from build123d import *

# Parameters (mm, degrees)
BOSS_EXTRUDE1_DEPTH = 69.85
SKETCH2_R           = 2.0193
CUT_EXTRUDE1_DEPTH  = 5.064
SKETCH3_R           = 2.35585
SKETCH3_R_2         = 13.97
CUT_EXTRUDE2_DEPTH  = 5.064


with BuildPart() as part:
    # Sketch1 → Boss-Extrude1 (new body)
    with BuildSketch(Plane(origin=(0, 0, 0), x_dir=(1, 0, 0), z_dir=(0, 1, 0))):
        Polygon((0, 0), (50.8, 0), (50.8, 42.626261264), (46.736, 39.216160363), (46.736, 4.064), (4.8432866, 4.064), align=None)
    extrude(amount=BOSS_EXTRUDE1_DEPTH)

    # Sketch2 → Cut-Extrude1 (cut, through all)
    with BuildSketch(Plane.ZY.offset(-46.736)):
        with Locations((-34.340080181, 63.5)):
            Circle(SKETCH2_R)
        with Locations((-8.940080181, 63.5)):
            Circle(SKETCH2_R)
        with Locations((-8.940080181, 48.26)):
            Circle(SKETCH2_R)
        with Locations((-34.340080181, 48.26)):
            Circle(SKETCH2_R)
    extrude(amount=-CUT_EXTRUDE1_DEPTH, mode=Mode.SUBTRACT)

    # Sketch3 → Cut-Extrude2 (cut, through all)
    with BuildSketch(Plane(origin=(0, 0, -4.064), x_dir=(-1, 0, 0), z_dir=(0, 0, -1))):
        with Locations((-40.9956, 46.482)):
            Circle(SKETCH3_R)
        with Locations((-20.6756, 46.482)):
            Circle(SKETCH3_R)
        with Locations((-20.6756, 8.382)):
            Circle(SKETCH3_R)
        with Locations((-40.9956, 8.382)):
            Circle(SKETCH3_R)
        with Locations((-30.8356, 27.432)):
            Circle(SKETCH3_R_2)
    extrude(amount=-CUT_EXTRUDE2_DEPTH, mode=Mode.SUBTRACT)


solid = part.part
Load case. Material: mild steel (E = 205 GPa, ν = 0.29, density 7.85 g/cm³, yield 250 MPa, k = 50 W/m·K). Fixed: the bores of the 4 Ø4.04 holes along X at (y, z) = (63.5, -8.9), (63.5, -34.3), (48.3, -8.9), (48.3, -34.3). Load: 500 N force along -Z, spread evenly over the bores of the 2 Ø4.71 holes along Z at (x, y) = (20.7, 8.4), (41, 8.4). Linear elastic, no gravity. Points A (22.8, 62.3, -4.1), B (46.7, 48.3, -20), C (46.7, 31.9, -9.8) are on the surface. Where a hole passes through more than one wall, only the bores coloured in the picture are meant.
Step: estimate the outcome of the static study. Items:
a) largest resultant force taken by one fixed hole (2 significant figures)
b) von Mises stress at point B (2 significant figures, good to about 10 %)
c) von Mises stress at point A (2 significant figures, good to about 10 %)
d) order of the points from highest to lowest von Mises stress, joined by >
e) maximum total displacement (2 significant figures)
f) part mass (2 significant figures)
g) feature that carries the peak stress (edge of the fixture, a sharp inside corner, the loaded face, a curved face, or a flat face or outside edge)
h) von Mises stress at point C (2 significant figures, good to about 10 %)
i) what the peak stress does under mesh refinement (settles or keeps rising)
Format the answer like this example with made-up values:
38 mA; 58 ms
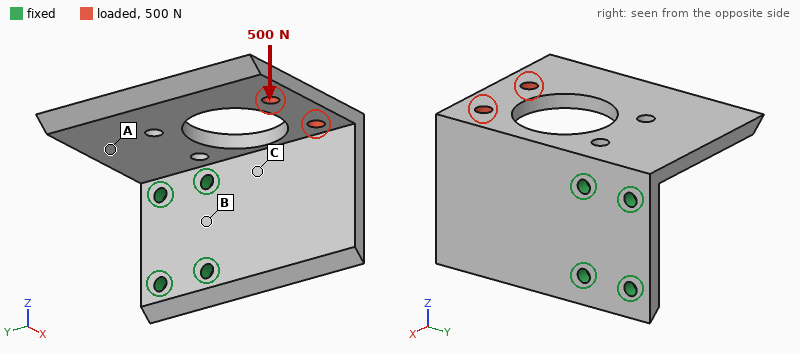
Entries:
720 N; 13 MPa; 29 MPa; C > A > B; 0.26 mm; 170 g; edge of the fixture; 44 MPa; keeps rising
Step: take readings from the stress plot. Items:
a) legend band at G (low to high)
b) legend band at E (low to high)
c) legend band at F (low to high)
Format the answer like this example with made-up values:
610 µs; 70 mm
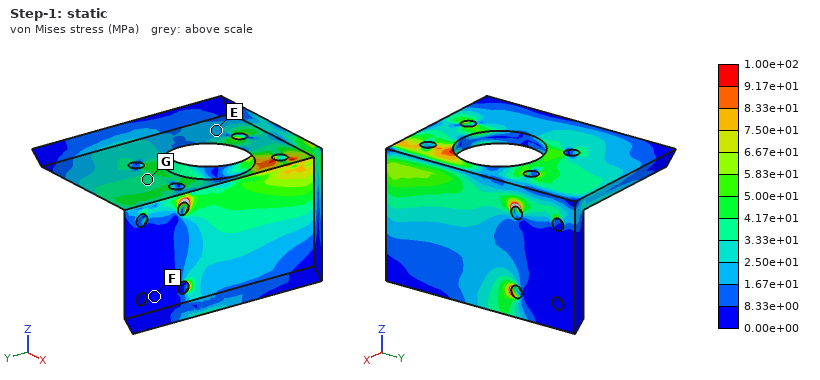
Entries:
3.33e+01 to 4.17e+01 MPa; 1.67e+01 to 2.50e+01 MPa; 0.00e+00 to 8.33e+00 MPa
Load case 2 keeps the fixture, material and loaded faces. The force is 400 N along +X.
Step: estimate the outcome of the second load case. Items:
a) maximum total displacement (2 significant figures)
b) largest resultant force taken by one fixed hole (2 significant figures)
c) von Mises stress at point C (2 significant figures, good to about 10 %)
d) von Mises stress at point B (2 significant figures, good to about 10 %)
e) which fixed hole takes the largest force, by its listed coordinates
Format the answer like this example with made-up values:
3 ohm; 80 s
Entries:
60 µm; 1.2 kN; 12 MPa; 12 MPa; (48.3, -8.9)
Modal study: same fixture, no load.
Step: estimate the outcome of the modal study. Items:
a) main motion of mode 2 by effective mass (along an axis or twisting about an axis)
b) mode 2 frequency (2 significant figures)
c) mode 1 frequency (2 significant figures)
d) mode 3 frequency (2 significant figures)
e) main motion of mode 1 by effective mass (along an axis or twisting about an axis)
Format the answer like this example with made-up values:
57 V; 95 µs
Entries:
along X; 2000 Hz; 1000 Hz; 2100 Hz; along Z
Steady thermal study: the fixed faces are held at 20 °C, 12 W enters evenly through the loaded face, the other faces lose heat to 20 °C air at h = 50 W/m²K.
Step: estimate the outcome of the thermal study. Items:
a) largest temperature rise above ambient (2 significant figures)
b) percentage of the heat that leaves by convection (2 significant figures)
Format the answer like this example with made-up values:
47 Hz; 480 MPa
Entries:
46 K; 64 %
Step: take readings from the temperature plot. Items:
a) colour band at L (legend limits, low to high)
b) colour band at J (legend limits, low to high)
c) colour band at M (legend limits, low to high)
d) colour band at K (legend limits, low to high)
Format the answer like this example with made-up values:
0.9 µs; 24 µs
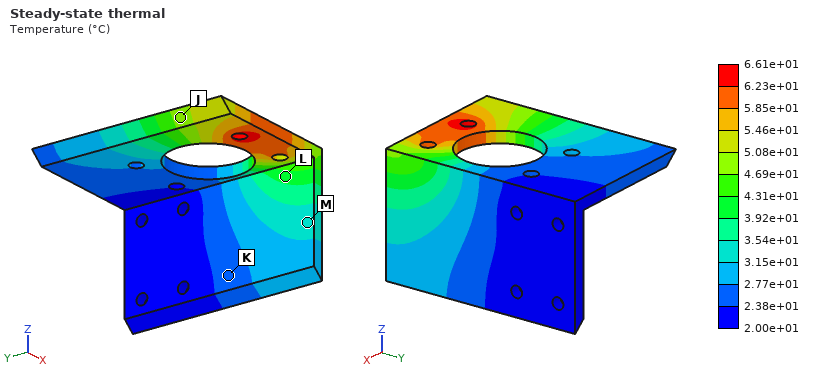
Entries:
3.92e+01 to 4.31e+01 °C; 4.69e+01 to 5.08e+01 °C; 3.15e+01 to 3.54e+01 °C; 2.38e+01 to 2.77e+01 °C
